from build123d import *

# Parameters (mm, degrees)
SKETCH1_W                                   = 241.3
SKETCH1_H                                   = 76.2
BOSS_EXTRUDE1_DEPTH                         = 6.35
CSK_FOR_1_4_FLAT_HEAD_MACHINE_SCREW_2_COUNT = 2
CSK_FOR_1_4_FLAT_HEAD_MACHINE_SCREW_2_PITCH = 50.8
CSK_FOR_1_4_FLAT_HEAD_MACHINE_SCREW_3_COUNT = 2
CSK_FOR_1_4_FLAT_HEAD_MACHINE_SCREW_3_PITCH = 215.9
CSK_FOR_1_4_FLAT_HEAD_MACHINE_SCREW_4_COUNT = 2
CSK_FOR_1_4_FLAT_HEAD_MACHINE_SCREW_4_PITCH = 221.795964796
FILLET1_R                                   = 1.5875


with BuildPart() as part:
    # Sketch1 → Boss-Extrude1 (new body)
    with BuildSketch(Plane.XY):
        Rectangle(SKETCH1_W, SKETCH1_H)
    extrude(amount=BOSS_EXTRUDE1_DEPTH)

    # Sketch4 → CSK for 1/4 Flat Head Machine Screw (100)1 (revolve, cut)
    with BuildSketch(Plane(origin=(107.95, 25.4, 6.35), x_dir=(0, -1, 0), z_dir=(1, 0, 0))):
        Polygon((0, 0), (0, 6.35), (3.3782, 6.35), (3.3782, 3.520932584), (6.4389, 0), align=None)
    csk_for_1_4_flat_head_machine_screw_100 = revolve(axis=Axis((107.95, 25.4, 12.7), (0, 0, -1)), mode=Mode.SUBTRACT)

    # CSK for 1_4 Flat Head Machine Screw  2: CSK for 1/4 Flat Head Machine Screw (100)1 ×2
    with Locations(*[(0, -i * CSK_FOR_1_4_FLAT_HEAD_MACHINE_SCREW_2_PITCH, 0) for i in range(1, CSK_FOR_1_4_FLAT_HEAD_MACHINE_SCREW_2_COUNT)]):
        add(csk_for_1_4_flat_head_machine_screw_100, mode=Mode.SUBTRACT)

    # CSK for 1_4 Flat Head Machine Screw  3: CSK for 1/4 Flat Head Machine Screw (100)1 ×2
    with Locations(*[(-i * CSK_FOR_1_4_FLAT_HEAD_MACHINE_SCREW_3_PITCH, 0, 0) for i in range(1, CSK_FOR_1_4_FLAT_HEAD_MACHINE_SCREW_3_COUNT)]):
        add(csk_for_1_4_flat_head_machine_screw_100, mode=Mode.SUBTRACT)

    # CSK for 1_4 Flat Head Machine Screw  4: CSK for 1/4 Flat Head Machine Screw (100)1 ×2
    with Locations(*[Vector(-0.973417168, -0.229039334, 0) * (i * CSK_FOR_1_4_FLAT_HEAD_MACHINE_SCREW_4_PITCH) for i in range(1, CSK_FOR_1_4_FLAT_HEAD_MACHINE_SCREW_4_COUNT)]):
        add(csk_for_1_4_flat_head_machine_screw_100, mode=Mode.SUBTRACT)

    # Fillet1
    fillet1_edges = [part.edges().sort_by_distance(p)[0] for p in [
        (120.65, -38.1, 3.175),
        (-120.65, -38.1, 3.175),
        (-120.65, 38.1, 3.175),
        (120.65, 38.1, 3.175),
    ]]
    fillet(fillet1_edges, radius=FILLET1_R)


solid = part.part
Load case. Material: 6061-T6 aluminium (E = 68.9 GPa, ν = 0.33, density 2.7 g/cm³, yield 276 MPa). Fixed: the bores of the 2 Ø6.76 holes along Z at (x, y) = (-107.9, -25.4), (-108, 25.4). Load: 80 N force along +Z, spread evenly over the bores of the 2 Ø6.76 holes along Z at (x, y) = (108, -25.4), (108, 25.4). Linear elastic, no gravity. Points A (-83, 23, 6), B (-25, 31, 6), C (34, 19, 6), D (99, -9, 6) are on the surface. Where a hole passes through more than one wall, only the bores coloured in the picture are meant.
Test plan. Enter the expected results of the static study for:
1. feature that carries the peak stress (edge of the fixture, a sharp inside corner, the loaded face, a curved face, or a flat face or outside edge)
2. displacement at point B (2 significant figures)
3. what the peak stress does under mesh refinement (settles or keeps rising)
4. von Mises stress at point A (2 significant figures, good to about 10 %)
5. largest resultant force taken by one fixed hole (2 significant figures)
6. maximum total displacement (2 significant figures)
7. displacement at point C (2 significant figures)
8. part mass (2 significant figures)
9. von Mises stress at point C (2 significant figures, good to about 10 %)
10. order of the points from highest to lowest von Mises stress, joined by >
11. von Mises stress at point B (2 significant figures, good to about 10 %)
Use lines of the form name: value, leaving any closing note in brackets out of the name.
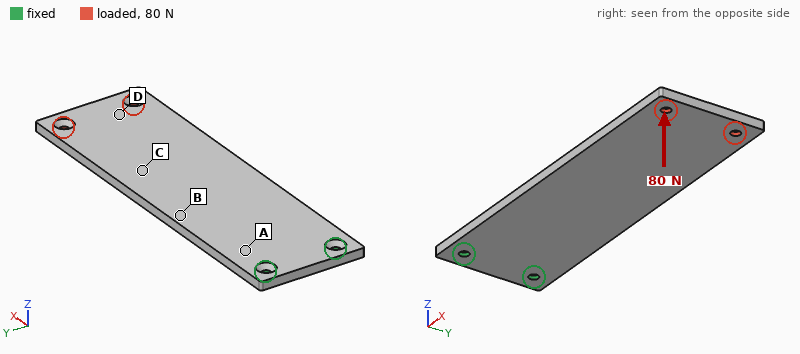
feature that carries the peak stress: edge of the fixture
displacement at point B: 0.59 mm
what the peak stress does under mesh refinement: keeps rising
von Mises stress at point A: 28 MPa
largest resultant force taken by one fixed hole: 130 N
maximum total displacement: 3.0 mm
displacement at point C: 1.4 mm
part mass: 310 g
von Mises stress at point C: 12 MPa
order of the points from highest to lowest von Mises stress, joined by >: A > B > C > D
von Mises stress at point B: 21 MPa
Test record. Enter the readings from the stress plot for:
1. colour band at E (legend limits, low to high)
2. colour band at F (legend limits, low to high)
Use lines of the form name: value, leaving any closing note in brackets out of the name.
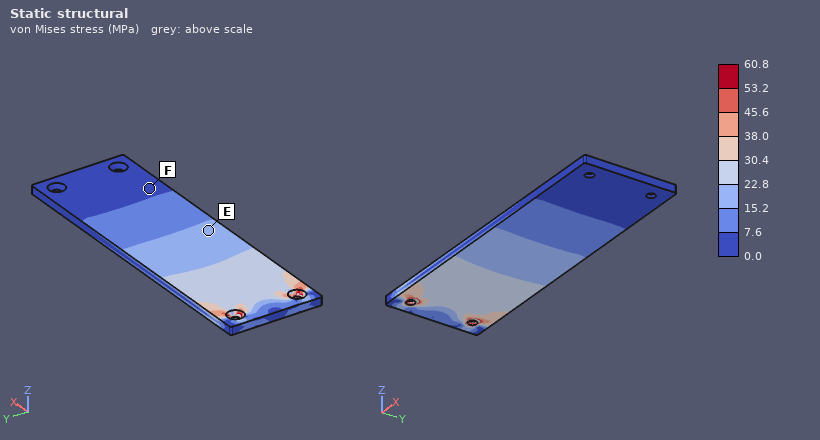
colour band at E: 15.2 to 22.8 MPa
colour band at F: 0.0 to 7.6 MPa
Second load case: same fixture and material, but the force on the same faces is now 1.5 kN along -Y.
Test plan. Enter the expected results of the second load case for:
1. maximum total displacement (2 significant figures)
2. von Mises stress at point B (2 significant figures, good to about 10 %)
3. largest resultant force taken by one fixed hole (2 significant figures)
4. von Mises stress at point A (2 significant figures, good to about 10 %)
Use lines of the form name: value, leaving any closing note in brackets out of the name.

maximum total displacement: 0.49 mm
von Mises stress at point B: 27 MPa
largest resultant force taken by one fixed hole: 6.1 kN
von Mises stress at point A: 27 MPa
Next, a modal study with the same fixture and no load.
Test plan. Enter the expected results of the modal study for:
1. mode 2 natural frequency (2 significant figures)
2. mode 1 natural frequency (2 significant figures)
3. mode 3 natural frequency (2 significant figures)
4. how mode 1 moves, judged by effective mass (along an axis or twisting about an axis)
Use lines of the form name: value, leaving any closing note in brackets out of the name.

mode 2 natural frequency: 580 Hz
mode 1 natural frequency: 92 Hz
mode 3 natural frequency: 590 Hz
how mode 1 moves, judged by effective mass: along Z
